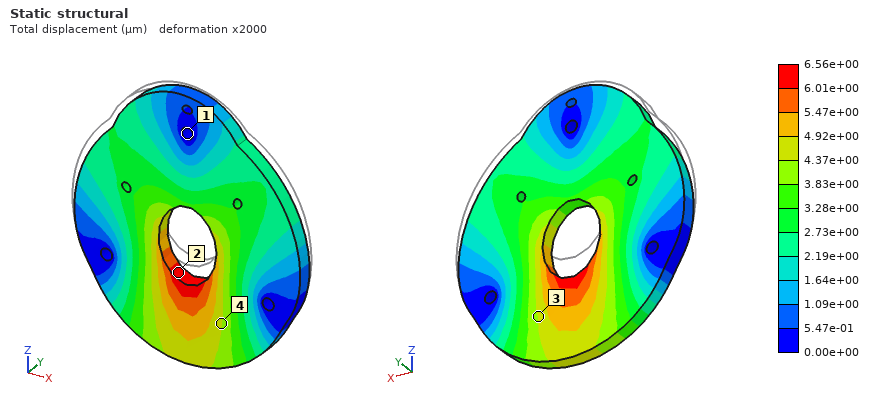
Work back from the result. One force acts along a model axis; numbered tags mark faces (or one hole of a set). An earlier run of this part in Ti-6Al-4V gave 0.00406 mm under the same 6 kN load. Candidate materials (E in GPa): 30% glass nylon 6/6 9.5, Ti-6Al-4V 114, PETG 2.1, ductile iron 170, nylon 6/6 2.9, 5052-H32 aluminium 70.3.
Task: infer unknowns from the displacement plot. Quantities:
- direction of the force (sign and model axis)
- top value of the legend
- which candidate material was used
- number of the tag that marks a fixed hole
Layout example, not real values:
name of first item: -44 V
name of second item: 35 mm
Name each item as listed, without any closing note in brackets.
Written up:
direction of the force: -Z
top value of the legend: 6.56e+00 µm
which candidate material was used: 5052-H32 aluminium
number of the tag that marks a fixed hole: 1
